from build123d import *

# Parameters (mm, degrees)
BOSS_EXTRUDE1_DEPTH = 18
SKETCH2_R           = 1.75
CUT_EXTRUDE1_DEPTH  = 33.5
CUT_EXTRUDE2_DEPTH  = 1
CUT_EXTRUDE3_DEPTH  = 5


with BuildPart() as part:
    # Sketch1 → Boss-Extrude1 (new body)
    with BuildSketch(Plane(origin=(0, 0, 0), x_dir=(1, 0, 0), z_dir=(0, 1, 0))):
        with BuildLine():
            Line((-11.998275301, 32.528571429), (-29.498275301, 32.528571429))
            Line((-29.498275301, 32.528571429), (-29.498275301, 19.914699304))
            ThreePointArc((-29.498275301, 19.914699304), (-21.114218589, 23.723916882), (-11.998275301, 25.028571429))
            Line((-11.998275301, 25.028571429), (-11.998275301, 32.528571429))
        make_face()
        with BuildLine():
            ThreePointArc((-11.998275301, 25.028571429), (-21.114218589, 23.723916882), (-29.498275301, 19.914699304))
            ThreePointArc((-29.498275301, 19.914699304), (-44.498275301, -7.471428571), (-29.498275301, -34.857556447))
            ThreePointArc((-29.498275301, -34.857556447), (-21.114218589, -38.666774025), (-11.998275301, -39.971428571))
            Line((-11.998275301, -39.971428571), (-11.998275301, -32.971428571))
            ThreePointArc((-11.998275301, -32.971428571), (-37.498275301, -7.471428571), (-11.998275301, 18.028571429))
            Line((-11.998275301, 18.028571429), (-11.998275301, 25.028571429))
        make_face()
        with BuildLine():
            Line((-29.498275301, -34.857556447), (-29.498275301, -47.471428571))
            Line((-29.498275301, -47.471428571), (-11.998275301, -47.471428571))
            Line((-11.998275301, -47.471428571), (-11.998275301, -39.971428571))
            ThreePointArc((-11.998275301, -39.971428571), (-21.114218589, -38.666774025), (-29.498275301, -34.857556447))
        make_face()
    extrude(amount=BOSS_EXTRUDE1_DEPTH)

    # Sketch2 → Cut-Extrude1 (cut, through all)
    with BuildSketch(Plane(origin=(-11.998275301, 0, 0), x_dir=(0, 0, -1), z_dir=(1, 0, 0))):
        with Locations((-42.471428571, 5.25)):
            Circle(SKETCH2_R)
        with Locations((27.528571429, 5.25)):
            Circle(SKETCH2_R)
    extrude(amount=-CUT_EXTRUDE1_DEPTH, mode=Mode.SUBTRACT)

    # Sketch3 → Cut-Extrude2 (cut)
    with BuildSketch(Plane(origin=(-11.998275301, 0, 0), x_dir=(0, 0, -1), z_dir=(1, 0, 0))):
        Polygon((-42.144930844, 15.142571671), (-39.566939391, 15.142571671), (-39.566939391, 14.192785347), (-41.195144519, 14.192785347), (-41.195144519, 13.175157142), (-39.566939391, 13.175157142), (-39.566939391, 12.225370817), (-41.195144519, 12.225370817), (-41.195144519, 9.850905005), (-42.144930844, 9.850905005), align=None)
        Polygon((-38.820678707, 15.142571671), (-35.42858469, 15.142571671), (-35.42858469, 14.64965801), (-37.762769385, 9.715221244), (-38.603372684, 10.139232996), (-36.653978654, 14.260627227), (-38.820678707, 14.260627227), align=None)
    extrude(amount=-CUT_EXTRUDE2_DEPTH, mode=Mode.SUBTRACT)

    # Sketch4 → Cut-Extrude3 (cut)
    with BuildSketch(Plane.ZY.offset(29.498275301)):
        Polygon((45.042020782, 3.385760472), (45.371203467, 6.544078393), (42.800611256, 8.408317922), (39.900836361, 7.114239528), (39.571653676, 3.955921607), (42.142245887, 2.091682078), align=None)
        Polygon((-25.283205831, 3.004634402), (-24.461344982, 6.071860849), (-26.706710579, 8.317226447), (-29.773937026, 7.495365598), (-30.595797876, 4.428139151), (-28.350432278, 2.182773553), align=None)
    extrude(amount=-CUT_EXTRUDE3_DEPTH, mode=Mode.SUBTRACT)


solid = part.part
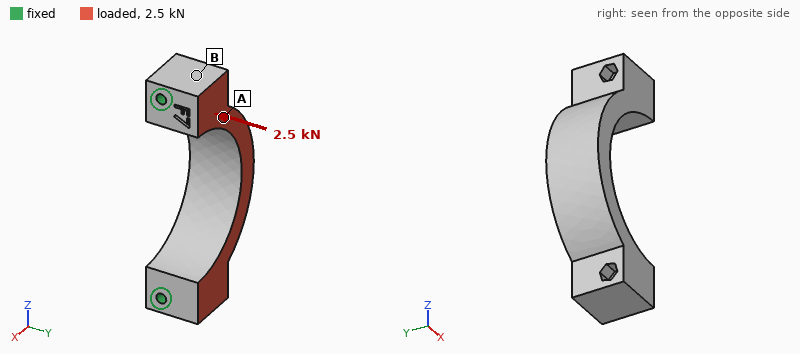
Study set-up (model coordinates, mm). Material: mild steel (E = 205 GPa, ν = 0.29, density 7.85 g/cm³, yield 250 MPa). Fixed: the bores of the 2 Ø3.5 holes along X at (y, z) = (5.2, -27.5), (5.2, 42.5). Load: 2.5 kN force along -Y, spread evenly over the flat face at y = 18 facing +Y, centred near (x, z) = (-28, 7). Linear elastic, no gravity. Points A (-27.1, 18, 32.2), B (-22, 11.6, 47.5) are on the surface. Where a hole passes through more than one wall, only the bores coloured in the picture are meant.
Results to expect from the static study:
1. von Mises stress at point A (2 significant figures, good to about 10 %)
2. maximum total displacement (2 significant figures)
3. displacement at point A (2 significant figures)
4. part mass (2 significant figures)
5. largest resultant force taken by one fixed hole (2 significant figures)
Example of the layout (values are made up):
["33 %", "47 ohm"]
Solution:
["16 MPa", "16 µm", "6.1 µm", "130 g", "1.3 kN"]
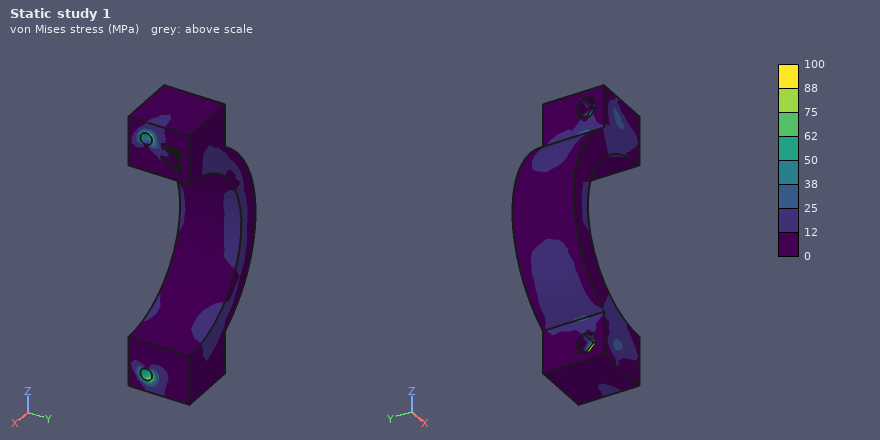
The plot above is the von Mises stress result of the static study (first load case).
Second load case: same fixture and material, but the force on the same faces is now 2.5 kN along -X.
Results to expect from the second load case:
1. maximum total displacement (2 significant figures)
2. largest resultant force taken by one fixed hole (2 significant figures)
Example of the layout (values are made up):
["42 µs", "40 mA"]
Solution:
["13 µm", "1.3 kN"]
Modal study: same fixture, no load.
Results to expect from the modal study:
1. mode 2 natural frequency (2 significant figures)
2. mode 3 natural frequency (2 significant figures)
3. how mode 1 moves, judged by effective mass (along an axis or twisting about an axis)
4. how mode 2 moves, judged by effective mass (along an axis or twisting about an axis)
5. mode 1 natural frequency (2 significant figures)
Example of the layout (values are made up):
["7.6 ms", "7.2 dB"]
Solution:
["13 kHz", "17 kHz", "along Y", "along Z", "6700 Hz"]
